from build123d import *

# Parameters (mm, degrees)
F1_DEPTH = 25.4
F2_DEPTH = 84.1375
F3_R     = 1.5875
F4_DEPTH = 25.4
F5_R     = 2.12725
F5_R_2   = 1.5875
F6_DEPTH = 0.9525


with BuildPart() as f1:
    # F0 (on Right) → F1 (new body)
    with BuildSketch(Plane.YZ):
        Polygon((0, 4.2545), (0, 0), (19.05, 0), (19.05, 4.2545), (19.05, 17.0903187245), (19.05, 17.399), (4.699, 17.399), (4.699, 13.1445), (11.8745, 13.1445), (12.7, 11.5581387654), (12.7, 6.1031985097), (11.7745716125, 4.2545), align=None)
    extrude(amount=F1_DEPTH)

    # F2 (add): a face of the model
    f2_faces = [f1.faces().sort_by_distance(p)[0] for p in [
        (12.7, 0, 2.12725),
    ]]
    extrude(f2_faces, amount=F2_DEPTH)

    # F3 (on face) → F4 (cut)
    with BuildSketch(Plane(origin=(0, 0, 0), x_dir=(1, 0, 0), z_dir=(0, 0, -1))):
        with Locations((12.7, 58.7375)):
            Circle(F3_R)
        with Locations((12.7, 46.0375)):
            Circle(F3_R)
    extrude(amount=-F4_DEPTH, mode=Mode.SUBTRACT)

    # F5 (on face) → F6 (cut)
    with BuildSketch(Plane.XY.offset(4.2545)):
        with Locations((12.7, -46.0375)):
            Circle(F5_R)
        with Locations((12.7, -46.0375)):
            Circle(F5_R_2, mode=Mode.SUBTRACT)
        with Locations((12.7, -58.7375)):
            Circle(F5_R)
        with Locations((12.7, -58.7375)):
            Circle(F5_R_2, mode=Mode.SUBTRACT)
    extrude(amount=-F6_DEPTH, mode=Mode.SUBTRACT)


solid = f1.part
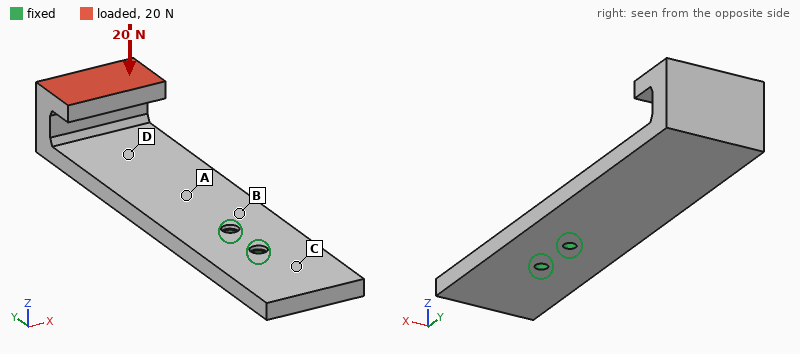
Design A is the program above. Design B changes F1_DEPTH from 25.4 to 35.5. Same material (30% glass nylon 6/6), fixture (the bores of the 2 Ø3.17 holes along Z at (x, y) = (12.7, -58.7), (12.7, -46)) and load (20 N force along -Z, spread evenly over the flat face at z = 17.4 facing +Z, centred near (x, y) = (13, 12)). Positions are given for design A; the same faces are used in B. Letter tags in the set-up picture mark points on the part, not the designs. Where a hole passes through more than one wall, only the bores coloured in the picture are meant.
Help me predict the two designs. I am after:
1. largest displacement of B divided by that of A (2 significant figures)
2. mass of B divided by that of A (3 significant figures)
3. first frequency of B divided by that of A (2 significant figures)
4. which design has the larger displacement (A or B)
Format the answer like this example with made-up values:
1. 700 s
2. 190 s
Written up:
1. 0.77
2. 1.40
3. 0.97
4. A
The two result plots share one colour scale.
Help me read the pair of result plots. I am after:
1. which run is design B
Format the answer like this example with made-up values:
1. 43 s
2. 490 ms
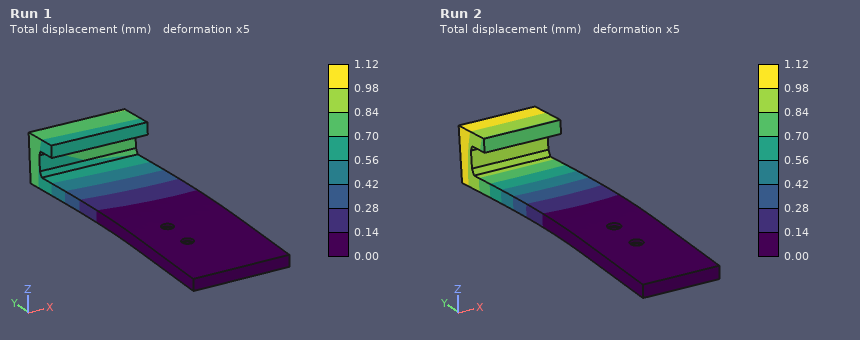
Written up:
1. Run 1
